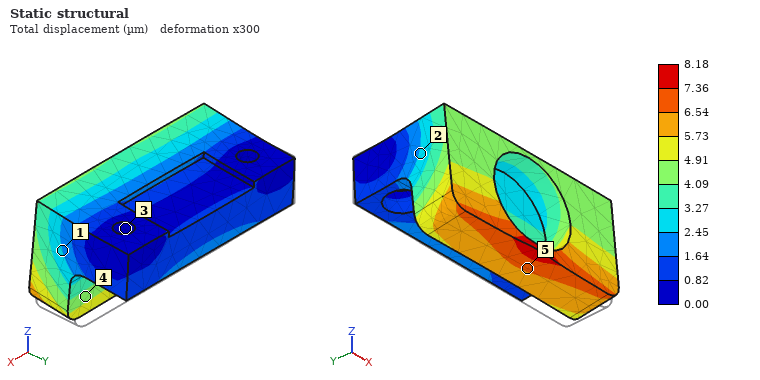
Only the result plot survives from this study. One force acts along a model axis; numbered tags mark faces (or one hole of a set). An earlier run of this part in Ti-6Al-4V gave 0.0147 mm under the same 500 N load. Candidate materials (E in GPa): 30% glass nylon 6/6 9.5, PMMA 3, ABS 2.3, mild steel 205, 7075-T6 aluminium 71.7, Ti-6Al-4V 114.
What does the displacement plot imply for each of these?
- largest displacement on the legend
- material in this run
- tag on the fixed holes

8.18 µm
mild steel
3
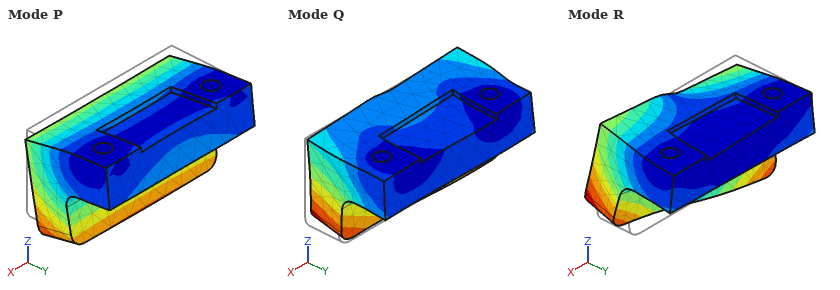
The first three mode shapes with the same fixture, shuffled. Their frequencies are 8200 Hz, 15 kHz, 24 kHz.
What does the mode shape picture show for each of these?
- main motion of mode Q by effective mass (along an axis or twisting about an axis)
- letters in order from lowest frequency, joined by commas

along X
P, R, Q
